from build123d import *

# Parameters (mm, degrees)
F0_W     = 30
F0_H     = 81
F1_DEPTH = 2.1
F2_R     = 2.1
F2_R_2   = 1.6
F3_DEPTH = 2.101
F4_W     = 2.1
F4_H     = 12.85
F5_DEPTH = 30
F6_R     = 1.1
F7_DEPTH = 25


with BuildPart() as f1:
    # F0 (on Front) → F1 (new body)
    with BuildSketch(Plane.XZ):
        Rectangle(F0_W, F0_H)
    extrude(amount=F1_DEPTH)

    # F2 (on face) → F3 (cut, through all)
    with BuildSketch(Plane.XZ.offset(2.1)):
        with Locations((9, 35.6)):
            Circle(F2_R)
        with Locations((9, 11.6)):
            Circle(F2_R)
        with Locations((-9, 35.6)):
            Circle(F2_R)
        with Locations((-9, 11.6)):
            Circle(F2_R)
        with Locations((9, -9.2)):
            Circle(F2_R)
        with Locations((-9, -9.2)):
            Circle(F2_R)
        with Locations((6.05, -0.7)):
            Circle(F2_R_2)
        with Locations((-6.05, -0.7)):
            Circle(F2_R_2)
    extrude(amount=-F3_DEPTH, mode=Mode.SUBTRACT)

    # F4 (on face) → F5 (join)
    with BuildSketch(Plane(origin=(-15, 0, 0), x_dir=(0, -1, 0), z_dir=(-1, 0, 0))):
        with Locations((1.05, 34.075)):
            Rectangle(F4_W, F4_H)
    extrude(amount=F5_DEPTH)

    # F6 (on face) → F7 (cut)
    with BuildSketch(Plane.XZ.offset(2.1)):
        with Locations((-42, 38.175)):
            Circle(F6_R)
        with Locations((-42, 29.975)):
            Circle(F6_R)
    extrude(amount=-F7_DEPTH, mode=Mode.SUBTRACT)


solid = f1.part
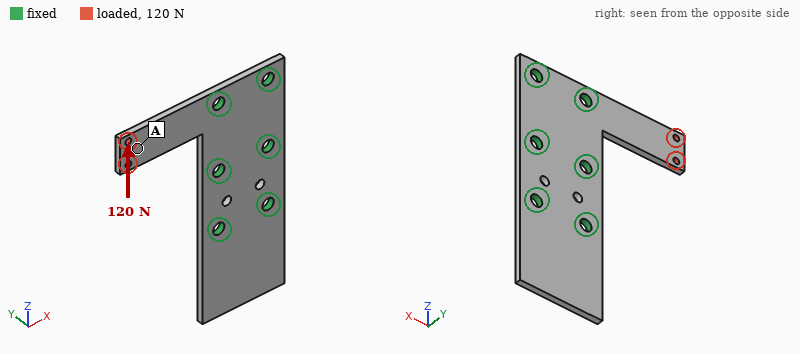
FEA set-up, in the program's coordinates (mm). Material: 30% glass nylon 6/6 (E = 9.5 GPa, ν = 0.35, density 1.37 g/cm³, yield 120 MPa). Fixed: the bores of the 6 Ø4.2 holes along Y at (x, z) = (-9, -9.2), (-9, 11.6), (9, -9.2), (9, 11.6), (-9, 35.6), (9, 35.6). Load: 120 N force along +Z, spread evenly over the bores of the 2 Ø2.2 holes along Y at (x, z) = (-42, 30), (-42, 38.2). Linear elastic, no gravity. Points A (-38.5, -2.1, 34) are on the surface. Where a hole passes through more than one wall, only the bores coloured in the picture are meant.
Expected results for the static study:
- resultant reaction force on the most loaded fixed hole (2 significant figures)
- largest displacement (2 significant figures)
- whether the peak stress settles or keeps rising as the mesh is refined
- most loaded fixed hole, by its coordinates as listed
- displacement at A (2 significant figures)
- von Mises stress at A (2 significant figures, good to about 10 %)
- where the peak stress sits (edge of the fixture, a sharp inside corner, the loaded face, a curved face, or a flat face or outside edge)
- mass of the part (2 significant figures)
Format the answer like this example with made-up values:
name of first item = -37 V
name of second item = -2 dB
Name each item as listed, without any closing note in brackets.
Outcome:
resultant reaction force on the most loaded fixed hole = 180 N
largest displacement = 0.50 mm
whether the peak stress settles or keeps rising as the mesh is refined = keeps rising
most loaded fixed hole, by its coordinates as listed = (-9, 35.6)
displacement at A = 0.36 mm
von Mises stress at A = 11 MPa
where the peak stress sits = a sharp inside corner
mass of the part = 7.8 g
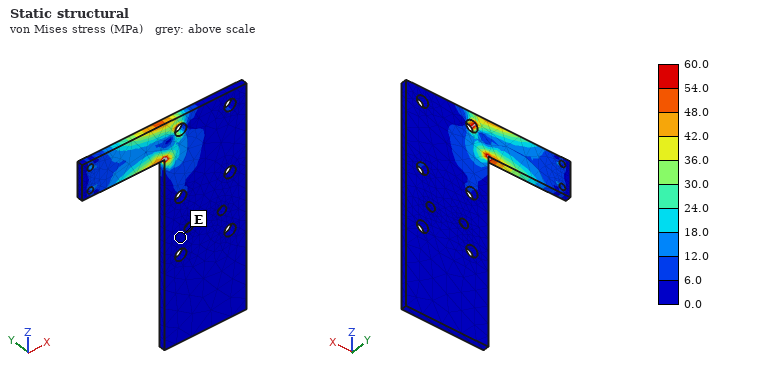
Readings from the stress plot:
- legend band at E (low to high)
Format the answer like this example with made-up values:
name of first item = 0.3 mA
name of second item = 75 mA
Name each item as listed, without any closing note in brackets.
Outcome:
legend band at E = 0.0 to 6.0 MPa
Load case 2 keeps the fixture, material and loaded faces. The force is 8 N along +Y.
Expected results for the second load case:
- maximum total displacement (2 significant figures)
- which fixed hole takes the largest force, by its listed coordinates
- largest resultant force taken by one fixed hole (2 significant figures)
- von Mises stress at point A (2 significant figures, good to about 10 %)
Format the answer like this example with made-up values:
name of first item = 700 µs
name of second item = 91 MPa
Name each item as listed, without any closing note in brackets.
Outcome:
maximum total displacement = 0.97 mm
which fixed hole takes the largest force, by its listed coordinates = (-9, 35.6)
largest resultant force taken by one fixed hole = 11 N
von Mises stress at point A = 3.2 MPa
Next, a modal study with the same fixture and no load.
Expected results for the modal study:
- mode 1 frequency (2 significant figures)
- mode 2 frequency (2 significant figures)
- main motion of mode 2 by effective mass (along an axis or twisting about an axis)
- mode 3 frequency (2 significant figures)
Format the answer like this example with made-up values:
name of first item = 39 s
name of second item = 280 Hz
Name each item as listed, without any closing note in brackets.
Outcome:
mode 1 frequency = 790 Hz
mode 2 frequency = 990 Hz
main motion of mode 2 by effective mass = along Y
mode 3 frequency = 2400 Hz
